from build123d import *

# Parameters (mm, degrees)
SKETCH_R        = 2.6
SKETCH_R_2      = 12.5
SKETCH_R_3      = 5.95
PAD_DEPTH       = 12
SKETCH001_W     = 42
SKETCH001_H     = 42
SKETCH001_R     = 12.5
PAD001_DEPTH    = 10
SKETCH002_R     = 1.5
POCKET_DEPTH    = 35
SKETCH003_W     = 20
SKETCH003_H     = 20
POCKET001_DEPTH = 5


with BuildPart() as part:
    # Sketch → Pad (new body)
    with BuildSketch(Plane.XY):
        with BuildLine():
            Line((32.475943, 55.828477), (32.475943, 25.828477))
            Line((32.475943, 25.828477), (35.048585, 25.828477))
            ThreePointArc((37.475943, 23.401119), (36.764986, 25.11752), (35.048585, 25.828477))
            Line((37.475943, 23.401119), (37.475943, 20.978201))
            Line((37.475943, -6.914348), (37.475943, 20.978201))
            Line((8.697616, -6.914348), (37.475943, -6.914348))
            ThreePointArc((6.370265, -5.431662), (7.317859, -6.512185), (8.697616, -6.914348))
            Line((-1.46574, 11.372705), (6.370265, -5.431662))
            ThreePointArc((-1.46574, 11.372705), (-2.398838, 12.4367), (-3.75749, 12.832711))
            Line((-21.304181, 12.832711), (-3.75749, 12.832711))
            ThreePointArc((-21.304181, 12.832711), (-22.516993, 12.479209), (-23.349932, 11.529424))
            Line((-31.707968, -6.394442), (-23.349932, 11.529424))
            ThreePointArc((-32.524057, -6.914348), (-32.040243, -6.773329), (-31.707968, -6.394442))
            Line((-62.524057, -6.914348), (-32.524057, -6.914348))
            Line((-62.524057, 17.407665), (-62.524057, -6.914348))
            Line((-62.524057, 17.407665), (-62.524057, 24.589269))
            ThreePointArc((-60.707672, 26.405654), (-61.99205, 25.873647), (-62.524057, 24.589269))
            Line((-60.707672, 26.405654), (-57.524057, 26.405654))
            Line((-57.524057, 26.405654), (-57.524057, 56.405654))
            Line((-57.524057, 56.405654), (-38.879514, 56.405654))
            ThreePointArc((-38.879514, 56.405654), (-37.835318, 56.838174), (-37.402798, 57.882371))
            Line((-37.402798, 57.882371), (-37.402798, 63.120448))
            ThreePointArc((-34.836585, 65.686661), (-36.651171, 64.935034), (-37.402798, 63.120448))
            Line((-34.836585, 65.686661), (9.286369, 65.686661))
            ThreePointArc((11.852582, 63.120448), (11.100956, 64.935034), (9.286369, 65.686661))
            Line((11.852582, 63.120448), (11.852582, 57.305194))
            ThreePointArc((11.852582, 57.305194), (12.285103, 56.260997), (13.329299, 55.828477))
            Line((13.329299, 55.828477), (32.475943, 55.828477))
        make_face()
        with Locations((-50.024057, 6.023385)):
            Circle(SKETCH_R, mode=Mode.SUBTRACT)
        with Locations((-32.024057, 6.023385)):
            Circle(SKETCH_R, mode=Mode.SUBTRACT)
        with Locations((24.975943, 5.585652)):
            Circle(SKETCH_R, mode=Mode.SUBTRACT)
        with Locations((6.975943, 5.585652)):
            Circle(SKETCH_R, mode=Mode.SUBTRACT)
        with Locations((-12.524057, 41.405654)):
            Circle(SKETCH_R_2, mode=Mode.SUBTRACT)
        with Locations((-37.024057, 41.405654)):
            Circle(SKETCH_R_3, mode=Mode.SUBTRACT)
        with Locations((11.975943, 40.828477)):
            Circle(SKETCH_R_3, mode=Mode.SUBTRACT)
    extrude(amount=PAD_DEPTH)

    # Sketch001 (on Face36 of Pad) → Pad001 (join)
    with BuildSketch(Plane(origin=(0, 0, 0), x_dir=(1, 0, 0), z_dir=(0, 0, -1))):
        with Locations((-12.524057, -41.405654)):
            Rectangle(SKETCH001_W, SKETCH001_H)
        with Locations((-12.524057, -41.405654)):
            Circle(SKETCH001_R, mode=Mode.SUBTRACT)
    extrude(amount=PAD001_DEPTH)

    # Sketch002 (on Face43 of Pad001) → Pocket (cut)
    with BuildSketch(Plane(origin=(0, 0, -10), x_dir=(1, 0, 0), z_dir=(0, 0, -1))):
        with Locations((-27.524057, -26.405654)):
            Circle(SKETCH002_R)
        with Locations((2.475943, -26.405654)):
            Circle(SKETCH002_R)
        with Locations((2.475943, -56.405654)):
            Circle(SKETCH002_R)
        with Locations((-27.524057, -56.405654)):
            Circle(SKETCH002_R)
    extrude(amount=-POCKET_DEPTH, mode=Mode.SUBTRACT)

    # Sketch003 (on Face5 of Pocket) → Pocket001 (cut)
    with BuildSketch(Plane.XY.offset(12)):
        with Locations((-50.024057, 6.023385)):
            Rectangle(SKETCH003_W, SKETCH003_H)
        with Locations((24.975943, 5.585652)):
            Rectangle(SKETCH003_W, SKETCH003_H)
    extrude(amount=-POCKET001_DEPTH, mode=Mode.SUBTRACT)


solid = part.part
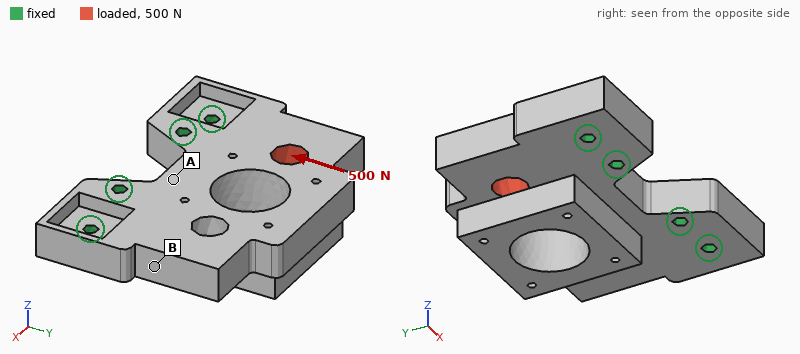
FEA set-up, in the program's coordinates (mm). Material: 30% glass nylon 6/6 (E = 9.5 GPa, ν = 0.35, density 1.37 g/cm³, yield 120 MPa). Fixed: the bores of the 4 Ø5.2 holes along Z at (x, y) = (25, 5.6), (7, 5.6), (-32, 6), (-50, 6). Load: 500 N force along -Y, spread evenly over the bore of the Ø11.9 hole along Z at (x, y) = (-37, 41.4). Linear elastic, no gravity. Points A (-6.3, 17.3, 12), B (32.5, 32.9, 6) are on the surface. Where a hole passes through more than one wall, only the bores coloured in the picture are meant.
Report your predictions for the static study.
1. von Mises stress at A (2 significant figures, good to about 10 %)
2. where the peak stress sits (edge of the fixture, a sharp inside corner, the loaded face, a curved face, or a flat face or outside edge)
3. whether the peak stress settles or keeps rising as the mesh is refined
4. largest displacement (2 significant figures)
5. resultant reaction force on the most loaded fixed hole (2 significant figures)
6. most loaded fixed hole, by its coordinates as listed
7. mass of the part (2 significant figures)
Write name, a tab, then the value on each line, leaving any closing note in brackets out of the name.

von Mises stress at A	0.51 MPa
where the peak stress sits	edge of the fixture
whether the peak stress settles or keeps rising as the mesh is refined	keeps rising
largest displacement	13 µm
resultant reaction force on the most loaded fixed hole	270 N
most loaded fixed hole, by its coordinates as listed	(-32, 6)
mass of the part	95 g
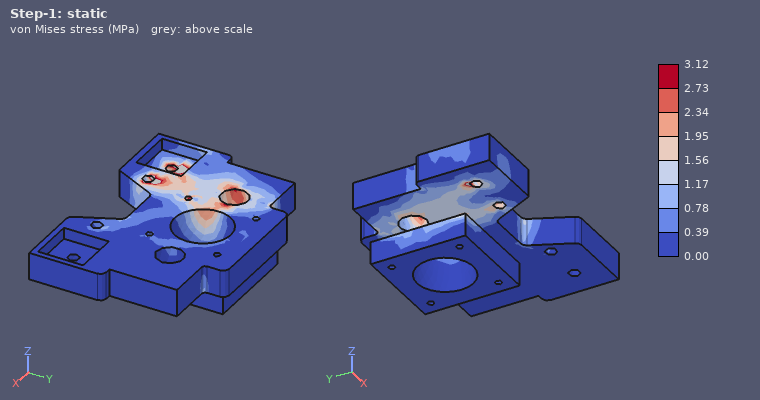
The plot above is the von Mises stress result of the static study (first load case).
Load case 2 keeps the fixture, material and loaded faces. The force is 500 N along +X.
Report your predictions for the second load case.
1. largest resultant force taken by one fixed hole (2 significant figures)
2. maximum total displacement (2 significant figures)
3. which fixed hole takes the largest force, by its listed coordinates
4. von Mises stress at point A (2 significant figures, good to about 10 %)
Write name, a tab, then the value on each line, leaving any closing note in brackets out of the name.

largest resultant force taken by one fixed hole	300 N
maximum total displacement	19 µm
which fixed hole takes the largest force, by its listed coordinates	(-50, 6)
von Mises stress at point A	1.7 MPa
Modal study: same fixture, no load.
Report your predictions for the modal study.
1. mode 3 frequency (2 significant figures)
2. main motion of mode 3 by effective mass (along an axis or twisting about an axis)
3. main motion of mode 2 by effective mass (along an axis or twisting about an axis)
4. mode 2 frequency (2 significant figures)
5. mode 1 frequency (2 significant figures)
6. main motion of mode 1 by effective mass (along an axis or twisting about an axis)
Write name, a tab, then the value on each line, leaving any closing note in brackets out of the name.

mode 3 frequency	4100 Hz
main motion of mode 3 by effective mass	along X
main motion of mode 2 by effective mass	twisting about Y
mode 2 frequency	2700 Hz
mode 1 frequency	1200 Hz
main motion of mode 1 by effective mass	along Z
